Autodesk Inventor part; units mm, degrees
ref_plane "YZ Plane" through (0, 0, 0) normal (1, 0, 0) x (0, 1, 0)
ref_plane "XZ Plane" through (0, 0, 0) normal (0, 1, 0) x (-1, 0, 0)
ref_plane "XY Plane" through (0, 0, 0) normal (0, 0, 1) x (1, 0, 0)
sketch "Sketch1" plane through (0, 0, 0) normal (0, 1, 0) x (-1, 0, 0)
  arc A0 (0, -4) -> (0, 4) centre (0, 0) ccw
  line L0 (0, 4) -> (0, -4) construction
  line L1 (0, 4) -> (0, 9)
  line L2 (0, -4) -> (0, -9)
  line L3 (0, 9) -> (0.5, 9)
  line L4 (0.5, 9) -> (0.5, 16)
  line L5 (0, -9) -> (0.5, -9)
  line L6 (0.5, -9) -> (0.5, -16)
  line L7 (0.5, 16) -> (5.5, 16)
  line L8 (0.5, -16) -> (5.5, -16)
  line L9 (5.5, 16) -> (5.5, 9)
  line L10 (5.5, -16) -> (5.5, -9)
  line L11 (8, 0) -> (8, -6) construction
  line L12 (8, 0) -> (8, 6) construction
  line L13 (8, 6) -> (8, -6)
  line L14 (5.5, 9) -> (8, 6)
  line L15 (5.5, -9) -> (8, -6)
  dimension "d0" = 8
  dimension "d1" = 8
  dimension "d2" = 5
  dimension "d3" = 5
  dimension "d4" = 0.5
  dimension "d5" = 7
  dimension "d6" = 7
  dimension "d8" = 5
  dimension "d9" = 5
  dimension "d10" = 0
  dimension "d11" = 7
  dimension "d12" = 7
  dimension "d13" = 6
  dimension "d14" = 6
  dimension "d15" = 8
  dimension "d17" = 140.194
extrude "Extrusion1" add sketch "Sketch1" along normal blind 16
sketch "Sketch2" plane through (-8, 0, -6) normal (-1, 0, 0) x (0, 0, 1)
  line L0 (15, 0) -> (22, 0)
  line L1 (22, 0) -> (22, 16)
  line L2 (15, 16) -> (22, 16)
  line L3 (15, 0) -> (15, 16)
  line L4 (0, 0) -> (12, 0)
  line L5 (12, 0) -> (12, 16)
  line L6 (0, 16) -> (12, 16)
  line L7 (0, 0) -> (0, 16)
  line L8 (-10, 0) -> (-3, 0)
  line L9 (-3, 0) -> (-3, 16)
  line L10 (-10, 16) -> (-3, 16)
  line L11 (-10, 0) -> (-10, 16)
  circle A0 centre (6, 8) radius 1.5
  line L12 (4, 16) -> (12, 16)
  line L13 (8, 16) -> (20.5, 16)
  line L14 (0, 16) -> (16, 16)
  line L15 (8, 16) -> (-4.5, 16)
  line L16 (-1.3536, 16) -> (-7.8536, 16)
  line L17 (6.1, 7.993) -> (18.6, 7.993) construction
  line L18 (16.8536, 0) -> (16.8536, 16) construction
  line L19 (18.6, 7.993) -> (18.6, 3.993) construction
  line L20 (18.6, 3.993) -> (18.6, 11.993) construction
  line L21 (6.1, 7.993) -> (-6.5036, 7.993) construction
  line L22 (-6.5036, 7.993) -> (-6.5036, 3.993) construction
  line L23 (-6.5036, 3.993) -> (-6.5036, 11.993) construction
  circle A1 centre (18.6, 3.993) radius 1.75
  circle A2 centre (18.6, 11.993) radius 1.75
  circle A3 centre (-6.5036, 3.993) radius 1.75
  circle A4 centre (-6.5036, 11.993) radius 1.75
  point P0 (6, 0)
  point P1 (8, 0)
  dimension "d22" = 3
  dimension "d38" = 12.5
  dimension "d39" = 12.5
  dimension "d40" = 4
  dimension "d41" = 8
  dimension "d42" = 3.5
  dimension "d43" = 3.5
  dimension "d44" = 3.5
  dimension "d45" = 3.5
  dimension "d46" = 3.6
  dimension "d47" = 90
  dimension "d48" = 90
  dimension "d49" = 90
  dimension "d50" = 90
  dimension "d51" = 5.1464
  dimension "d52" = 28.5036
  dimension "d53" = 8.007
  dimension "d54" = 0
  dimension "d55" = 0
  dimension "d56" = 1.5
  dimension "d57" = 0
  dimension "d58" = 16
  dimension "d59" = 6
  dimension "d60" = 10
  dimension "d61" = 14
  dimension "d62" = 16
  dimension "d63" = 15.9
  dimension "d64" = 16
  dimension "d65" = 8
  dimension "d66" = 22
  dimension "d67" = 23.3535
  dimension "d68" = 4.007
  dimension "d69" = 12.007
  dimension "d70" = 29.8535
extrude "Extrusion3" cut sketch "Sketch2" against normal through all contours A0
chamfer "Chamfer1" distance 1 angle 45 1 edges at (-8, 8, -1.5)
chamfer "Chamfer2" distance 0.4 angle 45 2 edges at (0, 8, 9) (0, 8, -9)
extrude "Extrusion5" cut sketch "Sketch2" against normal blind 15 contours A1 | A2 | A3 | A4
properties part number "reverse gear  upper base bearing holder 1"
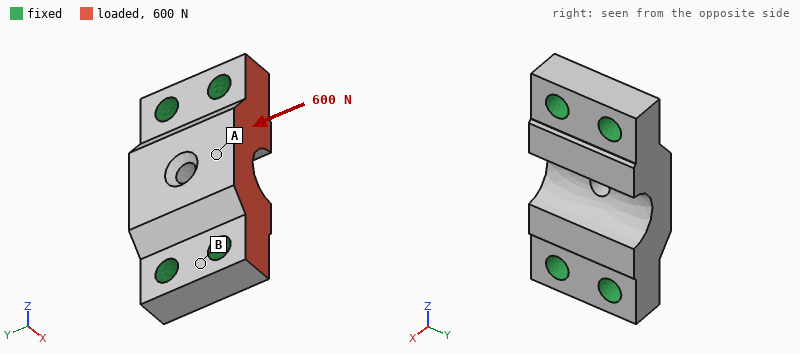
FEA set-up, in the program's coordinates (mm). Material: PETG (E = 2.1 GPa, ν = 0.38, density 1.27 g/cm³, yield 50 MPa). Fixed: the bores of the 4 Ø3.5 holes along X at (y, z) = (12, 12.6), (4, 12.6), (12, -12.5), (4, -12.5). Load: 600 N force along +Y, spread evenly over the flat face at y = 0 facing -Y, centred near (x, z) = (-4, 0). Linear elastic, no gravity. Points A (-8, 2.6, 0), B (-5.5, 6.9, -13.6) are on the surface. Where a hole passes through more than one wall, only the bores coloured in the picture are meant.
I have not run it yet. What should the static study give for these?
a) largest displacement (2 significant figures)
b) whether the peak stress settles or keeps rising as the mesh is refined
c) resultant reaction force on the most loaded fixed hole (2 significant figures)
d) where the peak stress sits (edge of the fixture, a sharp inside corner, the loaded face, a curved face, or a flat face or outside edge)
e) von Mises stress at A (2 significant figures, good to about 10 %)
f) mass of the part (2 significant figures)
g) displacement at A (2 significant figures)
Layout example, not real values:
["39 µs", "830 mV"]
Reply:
["57 µm", "keeps rising", "210 N", "edge of the fixture", "2.6 MPa", "3.4 g", "50 µm"]
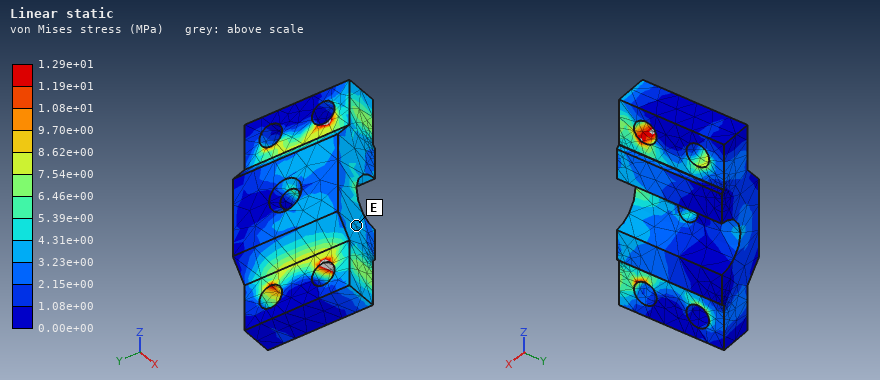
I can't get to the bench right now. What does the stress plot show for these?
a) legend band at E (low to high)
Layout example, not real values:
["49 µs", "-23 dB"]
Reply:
["3.23e+00 to 4.31e+00 MPa"]
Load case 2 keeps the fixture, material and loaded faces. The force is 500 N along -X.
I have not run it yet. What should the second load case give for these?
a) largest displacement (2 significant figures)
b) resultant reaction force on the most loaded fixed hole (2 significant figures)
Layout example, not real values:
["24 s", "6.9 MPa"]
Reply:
["0.15 mm", "290 N"]
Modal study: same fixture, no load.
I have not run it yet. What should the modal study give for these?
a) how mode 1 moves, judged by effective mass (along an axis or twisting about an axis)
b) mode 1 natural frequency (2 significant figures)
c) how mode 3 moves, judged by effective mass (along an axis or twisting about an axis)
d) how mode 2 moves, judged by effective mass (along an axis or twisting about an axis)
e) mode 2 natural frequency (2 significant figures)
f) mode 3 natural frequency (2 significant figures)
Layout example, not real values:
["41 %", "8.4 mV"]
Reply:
["along X", "10 kHz", "along Y", "along Y", "11 kHz", "15 kHz"]
